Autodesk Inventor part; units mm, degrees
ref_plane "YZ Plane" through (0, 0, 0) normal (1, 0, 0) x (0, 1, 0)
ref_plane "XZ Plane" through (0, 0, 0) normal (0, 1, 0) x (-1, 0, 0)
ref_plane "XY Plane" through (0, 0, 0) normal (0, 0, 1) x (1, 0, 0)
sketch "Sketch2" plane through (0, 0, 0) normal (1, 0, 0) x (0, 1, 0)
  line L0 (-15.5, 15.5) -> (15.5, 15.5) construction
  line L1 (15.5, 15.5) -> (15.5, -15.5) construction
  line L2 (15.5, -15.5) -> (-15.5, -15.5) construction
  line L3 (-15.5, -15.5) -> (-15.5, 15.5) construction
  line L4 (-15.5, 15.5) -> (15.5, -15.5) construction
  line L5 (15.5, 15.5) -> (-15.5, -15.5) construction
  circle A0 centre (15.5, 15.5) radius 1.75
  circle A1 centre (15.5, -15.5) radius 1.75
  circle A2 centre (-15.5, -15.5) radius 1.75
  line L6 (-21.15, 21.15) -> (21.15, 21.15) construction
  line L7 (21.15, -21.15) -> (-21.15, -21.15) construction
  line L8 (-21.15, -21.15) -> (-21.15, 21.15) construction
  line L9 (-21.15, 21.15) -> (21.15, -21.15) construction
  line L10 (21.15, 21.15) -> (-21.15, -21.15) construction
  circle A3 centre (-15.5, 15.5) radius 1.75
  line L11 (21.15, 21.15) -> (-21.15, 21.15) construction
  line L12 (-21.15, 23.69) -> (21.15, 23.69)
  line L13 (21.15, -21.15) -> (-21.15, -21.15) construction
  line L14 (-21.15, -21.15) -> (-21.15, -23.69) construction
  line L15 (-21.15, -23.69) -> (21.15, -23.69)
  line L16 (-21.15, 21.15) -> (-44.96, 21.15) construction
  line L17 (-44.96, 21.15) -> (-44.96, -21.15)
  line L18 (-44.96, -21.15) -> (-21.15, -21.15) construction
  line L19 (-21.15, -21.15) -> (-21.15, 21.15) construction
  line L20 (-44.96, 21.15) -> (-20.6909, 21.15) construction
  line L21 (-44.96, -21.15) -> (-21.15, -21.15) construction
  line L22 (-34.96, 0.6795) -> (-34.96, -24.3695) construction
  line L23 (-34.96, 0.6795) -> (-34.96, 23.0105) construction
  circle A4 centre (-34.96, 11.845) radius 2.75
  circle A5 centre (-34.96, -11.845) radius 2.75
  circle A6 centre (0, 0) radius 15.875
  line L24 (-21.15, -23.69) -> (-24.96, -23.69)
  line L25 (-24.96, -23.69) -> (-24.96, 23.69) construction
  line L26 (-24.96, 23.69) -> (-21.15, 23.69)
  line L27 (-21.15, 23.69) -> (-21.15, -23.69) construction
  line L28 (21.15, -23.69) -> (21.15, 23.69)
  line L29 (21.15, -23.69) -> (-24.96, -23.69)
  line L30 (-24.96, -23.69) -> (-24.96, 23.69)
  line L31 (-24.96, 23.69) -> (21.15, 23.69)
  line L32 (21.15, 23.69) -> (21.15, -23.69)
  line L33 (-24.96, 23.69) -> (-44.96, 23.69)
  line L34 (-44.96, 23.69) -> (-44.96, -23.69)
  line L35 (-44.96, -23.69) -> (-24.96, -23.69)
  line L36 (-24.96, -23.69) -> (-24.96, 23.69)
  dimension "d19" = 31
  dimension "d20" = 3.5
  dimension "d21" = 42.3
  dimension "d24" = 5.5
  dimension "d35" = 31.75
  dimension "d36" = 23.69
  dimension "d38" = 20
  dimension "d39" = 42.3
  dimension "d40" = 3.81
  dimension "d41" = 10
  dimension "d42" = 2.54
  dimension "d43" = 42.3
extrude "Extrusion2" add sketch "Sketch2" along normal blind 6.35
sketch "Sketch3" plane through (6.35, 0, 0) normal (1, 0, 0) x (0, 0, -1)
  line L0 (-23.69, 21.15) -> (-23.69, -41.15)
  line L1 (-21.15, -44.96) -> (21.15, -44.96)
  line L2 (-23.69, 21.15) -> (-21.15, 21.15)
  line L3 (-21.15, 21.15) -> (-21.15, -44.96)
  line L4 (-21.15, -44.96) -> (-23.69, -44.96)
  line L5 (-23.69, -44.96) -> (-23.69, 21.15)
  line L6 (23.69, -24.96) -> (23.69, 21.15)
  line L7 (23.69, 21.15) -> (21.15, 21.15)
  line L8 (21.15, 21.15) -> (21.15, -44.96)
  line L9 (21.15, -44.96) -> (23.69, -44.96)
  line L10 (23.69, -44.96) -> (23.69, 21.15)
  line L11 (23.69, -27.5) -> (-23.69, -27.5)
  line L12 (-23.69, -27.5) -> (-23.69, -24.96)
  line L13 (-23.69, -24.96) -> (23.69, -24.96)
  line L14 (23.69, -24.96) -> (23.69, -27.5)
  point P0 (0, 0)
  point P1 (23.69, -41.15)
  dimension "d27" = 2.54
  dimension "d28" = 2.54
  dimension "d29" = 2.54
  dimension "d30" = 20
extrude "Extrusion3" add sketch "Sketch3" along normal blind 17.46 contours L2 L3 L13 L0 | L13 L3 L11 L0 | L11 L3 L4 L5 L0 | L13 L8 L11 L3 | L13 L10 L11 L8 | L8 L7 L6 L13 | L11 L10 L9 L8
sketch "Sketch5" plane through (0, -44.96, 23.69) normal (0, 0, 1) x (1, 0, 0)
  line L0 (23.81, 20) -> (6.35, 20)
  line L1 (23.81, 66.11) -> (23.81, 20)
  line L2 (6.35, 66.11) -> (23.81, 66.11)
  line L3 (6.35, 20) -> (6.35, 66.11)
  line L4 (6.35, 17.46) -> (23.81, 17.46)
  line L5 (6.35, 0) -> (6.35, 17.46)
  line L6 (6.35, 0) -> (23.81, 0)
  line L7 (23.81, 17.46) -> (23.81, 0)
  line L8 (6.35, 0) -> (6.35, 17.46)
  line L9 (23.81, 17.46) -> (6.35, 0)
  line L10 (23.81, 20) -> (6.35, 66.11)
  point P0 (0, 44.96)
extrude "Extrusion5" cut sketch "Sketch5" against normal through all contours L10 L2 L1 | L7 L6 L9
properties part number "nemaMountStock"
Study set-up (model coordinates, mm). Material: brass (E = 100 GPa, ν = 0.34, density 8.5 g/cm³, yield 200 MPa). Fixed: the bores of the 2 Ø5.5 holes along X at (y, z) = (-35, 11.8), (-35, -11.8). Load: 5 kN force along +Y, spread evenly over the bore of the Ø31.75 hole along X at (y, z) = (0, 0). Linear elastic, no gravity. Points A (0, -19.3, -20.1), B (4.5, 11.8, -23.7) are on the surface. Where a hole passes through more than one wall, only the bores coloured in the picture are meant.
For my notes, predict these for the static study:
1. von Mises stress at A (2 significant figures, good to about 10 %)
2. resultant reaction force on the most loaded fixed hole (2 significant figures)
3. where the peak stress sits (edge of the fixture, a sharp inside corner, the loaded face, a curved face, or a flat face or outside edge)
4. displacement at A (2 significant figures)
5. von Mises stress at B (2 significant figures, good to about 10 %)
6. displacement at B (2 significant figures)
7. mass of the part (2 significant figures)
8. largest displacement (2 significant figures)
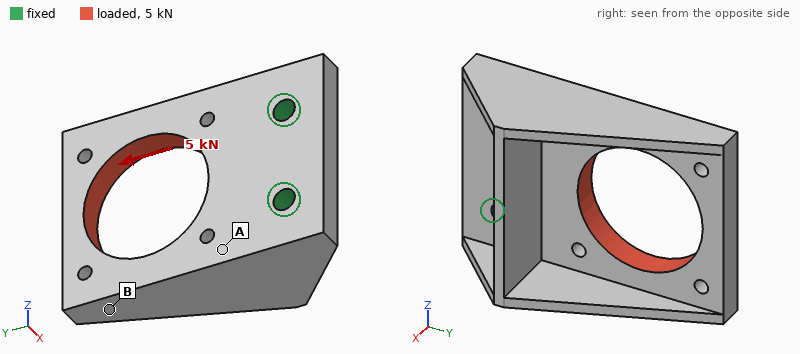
40 MPa
2.5 kN
a curved face
7.7 µm
12 MPa
18 µm
160 g
42 µm
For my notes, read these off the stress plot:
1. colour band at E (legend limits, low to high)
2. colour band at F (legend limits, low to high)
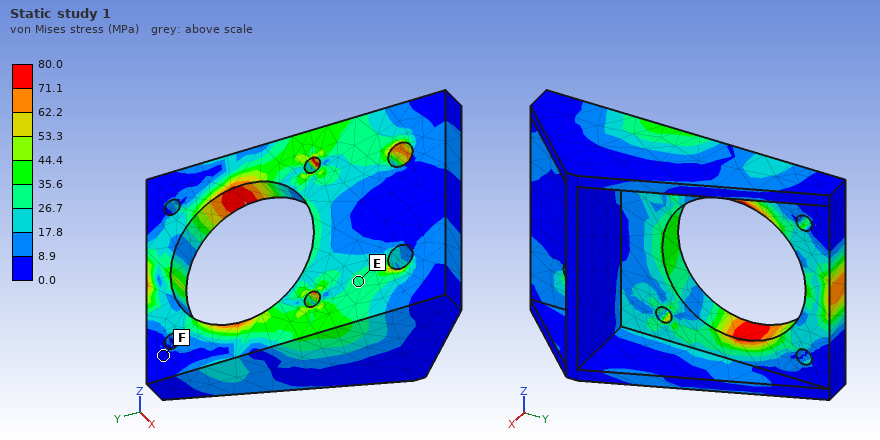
26.7 to 35.6 MPa
0.0 to 8.9 MPa
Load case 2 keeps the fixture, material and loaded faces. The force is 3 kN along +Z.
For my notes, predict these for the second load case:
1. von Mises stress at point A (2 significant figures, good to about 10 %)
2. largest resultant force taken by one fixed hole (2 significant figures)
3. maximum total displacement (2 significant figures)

39 MPa
3.9 kN
0.10 mm
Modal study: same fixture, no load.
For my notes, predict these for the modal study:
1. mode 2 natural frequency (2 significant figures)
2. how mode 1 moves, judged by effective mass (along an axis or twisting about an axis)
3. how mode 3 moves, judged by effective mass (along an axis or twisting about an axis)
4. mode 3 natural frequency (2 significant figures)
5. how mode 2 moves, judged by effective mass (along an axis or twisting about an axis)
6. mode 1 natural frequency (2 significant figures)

2500 Hz
along X
along Z
3800 Hz
twisting about Y
1800 Hz
